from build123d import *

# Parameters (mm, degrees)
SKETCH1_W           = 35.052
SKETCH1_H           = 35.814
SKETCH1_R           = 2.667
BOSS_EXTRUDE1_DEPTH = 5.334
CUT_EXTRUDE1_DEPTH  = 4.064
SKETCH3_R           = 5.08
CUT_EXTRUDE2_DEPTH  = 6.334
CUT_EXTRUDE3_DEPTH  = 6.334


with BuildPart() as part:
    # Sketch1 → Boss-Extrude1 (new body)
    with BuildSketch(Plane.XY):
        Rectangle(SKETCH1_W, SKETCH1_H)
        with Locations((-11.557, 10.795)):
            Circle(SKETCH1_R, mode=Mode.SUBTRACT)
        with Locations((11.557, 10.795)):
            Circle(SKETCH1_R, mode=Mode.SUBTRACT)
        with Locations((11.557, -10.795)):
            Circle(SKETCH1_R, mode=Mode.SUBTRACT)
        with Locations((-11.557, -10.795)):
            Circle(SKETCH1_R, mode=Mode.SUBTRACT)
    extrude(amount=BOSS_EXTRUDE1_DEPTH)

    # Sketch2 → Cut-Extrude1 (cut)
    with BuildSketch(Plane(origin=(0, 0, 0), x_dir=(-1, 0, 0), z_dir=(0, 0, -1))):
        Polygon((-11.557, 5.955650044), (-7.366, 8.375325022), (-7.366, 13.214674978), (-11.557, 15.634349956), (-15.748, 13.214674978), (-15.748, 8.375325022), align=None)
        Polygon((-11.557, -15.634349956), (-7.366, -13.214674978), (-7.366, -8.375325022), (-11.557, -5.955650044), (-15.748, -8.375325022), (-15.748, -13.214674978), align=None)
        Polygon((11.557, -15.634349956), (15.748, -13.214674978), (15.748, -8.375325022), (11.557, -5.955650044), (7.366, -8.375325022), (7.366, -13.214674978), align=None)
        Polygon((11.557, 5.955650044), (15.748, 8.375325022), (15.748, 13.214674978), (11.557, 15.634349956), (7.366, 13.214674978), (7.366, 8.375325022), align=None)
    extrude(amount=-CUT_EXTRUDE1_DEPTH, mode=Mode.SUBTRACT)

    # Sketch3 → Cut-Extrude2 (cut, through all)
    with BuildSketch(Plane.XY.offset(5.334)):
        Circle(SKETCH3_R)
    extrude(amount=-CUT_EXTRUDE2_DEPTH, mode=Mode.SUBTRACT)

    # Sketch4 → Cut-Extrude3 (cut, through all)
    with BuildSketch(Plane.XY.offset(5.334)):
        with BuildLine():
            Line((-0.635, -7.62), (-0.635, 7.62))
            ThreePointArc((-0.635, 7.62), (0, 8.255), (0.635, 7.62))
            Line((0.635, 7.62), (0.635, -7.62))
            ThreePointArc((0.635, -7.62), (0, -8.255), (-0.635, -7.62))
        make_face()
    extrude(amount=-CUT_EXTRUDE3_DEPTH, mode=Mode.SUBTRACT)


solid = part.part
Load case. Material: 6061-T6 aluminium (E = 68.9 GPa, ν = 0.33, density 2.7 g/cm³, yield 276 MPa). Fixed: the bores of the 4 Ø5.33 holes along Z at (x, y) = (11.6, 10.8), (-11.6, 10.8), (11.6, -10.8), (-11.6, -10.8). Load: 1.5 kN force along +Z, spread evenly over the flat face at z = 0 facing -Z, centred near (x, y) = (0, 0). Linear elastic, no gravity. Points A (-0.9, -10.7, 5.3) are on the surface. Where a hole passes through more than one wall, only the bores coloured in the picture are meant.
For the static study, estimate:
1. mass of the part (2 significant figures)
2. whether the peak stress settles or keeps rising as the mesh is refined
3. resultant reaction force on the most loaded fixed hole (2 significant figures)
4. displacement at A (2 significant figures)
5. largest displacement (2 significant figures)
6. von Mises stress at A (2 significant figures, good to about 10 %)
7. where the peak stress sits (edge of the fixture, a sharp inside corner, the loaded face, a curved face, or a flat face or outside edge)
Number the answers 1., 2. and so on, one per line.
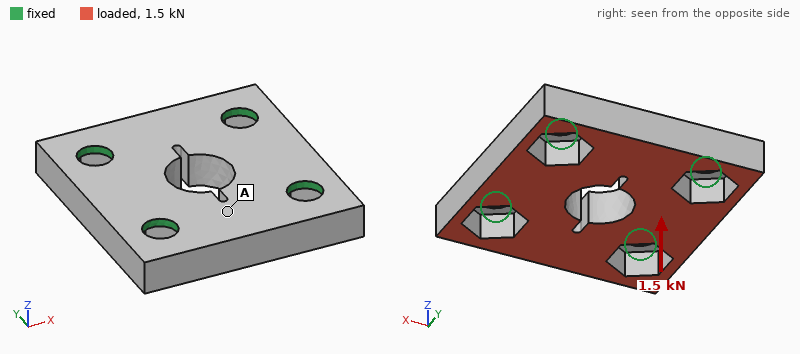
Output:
1. 14 g
2. keeps rising
3. 400 N
4. 4.9 µm
5. 6.0 µm
6. 8.7 MPa
7. edge of the fixture
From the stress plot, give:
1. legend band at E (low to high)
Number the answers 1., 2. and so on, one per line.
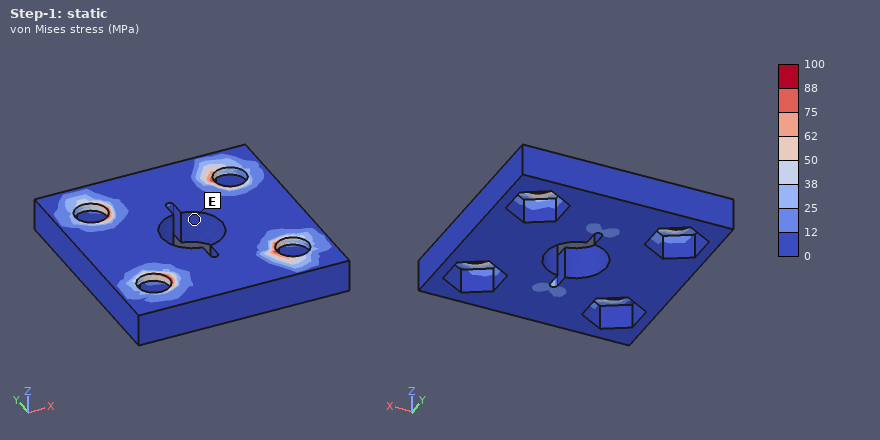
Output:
1. 0 to 12 MPa
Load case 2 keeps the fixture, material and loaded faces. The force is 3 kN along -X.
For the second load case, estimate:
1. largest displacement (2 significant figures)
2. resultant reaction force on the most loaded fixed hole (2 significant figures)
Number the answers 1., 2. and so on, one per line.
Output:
1. 10 µm
2. 800 N
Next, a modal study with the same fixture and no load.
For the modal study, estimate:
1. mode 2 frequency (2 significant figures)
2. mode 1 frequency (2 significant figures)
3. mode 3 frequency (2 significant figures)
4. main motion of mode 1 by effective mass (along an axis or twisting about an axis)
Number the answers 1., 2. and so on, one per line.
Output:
1. 26 kHz
2. 24 kHz
3. 28 kHz
4. along Z
